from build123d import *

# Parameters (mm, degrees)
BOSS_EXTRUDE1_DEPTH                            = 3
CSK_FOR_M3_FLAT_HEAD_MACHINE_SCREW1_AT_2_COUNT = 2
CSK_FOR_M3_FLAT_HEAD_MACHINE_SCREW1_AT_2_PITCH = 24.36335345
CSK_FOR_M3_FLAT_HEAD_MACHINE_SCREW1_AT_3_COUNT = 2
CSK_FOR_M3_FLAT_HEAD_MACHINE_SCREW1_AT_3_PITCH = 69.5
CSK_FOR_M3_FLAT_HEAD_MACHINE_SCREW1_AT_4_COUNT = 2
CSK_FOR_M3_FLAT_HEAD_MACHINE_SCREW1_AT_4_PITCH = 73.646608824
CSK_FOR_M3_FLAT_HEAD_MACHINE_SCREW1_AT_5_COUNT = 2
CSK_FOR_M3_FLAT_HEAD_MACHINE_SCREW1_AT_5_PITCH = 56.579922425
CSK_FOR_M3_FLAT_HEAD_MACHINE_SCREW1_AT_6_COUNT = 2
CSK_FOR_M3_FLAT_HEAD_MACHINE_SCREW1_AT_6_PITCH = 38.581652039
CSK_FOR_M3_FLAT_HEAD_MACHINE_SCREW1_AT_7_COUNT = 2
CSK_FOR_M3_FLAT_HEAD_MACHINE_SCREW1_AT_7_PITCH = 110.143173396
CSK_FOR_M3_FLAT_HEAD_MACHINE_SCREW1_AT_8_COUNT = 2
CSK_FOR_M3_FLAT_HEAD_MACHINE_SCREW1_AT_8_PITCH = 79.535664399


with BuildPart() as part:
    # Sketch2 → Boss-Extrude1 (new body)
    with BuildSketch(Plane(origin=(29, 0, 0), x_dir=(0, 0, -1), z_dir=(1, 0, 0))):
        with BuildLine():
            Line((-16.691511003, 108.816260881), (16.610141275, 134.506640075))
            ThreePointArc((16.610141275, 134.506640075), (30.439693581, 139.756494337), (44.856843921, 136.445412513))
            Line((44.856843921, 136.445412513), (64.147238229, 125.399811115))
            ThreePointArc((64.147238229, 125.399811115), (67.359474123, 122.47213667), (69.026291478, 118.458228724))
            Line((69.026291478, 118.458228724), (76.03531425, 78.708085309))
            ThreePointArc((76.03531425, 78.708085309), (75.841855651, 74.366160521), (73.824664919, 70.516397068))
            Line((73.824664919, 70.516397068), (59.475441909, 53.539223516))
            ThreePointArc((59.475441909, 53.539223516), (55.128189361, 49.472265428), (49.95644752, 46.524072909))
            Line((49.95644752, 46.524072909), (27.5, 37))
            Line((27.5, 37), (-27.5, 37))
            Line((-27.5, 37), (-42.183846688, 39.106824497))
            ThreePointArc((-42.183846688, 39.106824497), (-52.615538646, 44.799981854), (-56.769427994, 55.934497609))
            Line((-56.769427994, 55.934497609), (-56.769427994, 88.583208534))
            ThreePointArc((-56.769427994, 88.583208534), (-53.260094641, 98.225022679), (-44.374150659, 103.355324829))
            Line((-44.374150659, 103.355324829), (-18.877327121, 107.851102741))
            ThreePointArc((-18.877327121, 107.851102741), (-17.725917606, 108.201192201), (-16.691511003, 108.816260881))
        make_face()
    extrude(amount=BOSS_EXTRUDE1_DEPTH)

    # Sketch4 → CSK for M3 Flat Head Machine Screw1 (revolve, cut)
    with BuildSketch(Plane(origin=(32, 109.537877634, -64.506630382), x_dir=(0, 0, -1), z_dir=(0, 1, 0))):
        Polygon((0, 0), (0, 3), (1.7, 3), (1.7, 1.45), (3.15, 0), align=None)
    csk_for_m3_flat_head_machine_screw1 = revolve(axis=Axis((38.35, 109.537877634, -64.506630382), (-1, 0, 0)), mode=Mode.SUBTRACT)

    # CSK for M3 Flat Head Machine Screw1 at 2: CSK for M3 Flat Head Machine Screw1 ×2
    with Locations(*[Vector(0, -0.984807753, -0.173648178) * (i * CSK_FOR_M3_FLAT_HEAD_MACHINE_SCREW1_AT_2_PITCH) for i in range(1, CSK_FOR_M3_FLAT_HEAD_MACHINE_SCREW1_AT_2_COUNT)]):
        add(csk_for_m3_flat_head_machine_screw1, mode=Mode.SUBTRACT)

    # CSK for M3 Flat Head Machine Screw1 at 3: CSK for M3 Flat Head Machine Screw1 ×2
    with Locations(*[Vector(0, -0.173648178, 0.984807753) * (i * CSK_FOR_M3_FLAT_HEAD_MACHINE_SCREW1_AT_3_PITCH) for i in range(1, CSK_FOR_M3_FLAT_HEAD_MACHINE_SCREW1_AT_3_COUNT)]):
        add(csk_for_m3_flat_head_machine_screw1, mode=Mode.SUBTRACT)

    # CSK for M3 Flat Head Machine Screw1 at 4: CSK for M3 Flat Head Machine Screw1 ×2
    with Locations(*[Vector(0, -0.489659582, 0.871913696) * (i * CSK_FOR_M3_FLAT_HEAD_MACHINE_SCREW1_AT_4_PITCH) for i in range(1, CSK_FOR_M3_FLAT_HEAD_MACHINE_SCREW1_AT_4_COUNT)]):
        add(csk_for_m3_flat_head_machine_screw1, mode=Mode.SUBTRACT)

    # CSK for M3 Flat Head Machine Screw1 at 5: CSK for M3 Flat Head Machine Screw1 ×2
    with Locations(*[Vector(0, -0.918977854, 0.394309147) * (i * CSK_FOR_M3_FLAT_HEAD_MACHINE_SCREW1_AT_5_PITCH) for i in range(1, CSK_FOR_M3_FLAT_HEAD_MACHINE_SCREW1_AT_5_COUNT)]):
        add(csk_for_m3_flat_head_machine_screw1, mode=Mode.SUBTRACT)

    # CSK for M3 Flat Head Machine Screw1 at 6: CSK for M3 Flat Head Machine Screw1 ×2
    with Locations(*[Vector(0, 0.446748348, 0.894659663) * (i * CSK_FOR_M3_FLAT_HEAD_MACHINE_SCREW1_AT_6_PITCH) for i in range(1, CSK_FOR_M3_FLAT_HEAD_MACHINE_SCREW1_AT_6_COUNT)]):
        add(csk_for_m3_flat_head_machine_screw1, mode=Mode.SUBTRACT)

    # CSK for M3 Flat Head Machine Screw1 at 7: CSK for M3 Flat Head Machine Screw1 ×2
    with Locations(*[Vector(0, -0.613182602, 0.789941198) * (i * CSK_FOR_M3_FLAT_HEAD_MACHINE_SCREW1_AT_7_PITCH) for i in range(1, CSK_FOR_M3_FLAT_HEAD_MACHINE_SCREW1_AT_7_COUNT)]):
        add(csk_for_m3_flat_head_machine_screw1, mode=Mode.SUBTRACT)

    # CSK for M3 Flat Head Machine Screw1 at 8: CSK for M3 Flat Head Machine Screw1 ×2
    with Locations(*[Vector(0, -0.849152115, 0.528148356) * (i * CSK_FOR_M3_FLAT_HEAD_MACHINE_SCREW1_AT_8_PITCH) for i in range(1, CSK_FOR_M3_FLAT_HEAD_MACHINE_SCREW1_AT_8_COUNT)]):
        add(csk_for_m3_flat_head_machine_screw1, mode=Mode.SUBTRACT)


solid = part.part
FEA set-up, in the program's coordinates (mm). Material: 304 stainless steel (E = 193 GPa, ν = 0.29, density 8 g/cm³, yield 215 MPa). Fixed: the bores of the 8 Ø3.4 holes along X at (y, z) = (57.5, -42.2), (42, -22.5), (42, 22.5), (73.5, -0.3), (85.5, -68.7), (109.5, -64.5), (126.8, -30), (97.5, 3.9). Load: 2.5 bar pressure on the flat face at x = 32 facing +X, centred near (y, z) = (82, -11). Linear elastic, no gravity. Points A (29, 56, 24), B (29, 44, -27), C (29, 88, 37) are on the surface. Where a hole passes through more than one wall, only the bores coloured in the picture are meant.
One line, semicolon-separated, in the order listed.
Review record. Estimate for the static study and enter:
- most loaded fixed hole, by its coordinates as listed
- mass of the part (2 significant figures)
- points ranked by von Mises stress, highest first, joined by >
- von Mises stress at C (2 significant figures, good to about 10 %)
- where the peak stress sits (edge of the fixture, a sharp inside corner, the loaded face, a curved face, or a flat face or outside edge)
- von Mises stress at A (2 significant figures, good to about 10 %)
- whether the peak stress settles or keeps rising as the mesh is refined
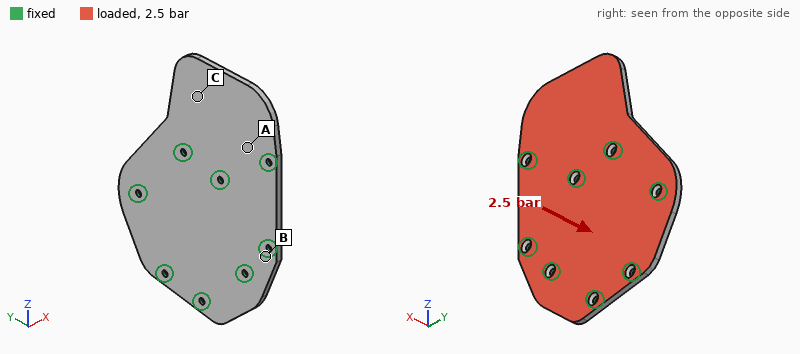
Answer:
(97.5, 3.9); 240 g; A > C > B; 33 MPa; edge of the fixture; 85 MPa; keeps rising
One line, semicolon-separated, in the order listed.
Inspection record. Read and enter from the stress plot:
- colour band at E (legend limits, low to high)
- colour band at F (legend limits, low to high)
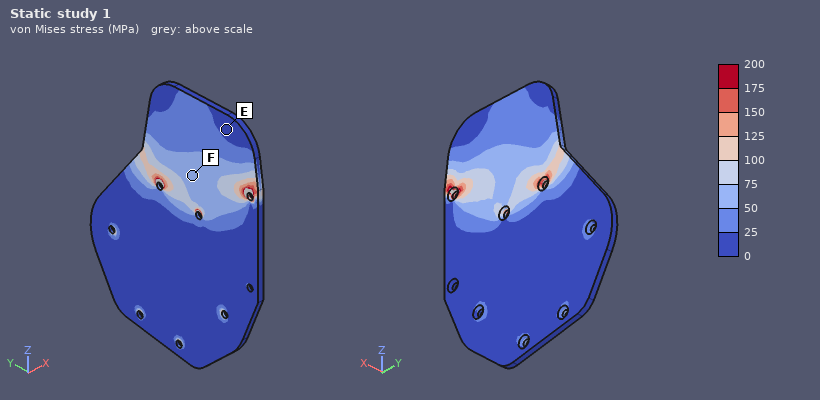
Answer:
0 to 25 MPa; 50 to 75 MPa
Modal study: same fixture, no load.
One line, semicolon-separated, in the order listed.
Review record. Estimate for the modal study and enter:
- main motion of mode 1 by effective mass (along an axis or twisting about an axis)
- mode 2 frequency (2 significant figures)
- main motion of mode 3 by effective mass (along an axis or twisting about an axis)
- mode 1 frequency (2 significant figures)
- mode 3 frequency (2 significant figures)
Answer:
along X; 2800 Hz; along X; 1100 Hz; 4100 Hz
